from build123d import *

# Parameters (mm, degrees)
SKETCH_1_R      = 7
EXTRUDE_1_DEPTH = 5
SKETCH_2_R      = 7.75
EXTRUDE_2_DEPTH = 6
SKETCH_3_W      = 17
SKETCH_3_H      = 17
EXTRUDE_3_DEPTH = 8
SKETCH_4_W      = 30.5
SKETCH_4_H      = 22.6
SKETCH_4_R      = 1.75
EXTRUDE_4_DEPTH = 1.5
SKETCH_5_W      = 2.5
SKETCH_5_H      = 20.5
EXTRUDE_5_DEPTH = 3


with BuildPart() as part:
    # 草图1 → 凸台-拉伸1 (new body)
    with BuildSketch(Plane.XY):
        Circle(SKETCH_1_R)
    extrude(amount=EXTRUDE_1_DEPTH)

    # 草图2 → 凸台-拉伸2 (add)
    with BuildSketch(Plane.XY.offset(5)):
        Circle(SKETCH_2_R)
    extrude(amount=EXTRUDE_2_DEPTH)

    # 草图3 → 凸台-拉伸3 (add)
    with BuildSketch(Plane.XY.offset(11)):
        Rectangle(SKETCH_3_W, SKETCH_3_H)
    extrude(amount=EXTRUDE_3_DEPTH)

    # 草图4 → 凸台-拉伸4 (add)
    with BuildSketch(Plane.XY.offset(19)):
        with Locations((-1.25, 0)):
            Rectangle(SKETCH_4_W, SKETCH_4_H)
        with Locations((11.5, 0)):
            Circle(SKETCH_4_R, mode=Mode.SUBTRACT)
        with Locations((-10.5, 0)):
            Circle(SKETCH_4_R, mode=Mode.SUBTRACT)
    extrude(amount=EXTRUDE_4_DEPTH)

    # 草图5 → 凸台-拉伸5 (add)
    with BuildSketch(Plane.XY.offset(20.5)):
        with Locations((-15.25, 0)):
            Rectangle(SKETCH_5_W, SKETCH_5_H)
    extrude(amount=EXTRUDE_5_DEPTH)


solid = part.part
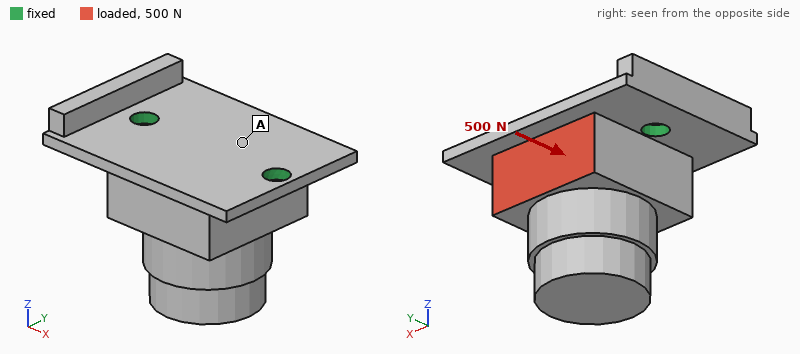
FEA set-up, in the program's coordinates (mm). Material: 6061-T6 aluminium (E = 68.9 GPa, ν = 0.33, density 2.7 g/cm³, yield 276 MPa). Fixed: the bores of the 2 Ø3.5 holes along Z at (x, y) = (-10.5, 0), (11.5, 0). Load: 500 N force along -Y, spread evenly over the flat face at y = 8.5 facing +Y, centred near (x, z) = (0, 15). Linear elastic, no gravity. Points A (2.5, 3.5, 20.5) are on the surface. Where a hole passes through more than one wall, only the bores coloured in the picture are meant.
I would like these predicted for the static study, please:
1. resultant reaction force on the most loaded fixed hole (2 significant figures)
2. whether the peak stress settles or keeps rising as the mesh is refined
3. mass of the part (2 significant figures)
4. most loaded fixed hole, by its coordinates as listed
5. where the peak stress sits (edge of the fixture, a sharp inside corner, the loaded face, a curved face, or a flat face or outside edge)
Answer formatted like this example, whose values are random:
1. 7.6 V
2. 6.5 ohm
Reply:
1. 270 N
2. keeps rising
3. 15 g
4. (-10.5, 0)
5. edge of the fixture
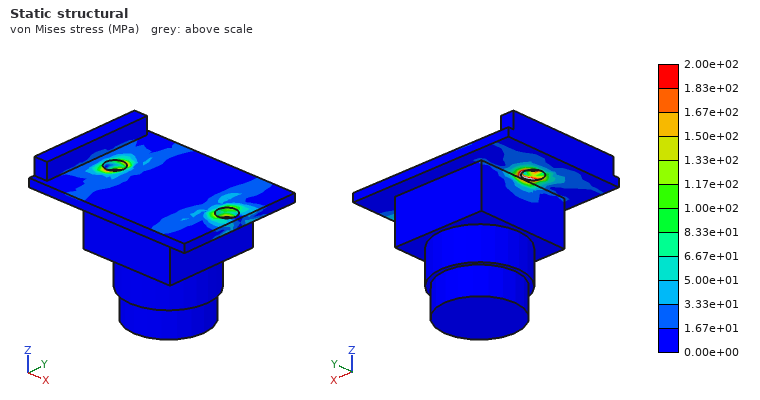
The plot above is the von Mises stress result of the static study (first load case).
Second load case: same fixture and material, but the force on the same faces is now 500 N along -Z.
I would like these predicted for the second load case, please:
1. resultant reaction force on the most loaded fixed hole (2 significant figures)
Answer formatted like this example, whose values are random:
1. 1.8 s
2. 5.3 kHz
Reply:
1. 290 N
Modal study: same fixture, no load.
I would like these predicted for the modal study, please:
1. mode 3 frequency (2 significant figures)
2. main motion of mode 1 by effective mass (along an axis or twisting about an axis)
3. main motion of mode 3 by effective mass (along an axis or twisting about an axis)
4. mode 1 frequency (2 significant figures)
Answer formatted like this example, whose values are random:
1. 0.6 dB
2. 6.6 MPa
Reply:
1. 17 kHz
2. along Y
3. along Z
4. 3500 Hz
